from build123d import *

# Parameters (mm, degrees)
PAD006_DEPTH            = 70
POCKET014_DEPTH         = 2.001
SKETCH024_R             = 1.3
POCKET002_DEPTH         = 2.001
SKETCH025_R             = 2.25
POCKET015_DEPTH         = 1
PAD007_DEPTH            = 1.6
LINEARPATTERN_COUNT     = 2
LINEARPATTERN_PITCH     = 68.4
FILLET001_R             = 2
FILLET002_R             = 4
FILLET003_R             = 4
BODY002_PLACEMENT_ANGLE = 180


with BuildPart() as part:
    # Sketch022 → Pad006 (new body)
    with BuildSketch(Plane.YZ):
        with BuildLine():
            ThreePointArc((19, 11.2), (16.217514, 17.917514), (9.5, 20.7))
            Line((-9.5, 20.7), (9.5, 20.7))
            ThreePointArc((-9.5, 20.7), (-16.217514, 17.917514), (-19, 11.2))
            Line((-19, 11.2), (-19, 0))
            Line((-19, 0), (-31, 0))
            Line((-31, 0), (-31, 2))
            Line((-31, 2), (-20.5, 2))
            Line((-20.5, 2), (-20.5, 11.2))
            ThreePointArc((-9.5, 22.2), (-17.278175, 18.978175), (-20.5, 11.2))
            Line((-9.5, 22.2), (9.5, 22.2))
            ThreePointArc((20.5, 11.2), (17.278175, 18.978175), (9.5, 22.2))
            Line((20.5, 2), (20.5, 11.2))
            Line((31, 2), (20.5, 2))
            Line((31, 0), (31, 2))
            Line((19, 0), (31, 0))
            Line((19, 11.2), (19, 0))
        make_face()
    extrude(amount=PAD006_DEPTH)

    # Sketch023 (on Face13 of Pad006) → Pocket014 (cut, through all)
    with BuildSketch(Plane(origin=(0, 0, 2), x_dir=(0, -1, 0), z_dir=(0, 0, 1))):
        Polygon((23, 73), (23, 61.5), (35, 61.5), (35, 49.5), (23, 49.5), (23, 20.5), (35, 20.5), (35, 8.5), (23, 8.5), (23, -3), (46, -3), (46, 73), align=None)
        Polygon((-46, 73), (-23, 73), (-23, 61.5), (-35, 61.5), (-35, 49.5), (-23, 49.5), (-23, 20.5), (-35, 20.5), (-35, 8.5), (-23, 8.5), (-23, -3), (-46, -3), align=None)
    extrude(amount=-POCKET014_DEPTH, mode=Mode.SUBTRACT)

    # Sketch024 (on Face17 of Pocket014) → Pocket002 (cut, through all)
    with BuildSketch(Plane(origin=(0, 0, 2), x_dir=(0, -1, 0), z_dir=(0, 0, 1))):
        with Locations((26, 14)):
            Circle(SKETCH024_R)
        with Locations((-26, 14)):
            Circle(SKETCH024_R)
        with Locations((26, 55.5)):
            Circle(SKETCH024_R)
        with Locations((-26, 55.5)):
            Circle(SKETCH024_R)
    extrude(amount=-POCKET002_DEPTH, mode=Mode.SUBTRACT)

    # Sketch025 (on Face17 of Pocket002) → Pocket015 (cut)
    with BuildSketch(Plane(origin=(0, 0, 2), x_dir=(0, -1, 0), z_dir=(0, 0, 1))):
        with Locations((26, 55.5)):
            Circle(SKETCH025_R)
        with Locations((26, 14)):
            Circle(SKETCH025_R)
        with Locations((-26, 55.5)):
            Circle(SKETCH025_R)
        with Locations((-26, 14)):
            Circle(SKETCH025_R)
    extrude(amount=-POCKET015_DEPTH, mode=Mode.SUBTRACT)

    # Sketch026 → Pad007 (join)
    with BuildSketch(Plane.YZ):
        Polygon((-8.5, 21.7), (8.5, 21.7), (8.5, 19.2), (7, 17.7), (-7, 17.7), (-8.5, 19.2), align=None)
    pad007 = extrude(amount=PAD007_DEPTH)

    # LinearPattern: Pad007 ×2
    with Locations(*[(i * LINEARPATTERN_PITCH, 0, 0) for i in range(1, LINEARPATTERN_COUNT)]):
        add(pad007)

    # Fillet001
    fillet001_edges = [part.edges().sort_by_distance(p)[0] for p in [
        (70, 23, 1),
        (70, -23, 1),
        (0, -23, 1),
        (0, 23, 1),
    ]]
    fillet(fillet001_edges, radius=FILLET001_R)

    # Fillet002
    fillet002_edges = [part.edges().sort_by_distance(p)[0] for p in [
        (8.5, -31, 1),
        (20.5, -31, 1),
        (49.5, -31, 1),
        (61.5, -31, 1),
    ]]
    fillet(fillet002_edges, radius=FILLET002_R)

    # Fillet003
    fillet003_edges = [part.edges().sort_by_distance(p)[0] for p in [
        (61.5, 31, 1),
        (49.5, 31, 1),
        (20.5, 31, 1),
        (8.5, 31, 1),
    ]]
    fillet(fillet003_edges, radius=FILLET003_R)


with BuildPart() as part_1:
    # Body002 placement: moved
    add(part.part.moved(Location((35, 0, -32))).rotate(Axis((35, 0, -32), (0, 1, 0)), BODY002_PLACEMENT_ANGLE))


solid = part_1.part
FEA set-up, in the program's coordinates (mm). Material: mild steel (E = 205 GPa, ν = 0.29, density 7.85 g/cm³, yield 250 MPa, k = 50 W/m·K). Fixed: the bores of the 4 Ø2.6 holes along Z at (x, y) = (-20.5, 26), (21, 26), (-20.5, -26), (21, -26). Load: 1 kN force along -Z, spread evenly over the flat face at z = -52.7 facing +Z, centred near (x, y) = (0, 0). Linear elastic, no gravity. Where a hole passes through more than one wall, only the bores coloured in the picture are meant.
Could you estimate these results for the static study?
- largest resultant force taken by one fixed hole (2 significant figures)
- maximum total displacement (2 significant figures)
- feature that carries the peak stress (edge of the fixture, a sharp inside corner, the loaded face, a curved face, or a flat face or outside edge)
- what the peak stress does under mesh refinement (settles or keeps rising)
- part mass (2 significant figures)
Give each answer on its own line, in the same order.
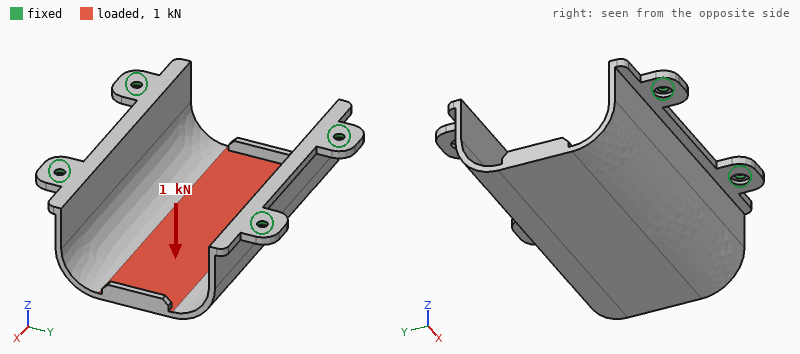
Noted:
300 N
66 µm
edge of the fixture
keeps rising
72 g
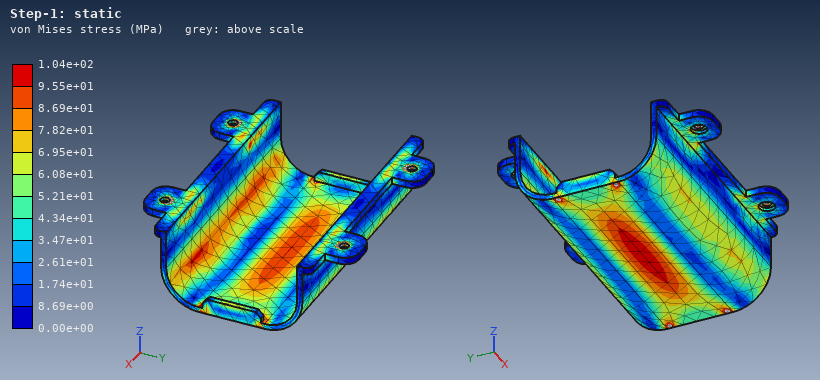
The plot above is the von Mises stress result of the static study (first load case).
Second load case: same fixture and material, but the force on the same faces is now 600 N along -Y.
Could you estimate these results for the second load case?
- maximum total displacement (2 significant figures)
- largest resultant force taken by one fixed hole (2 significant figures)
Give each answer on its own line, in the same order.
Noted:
0.11 mm
180 N
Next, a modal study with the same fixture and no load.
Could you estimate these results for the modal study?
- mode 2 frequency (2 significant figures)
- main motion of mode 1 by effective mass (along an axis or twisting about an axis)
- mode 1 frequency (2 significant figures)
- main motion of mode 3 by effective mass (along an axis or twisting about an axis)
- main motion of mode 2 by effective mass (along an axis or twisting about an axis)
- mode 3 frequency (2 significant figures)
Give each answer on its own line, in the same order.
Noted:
3500 Hz
along Y
1900 Hz
along X
twisting about Z
4200 Hz
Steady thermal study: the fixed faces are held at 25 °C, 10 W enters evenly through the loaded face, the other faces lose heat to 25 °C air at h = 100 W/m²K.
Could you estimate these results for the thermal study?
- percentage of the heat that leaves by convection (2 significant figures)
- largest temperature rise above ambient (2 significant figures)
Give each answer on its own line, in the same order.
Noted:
84 %
18 K
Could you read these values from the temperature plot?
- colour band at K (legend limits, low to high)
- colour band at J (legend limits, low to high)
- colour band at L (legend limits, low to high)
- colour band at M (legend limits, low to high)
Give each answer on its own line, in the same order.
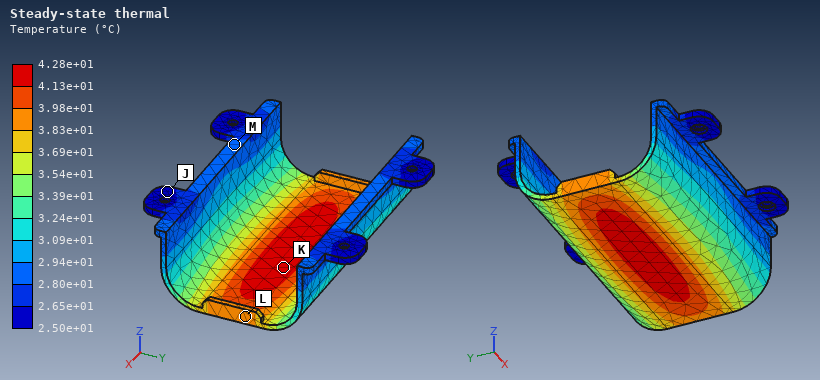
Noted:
4.13e+01 to 4.28e+01 °C
2.50e+01 to 2.65e+01 °C
3.83e+01 to 3.98e+01 °C
2.80e+01 to 2.94e+01 °C
